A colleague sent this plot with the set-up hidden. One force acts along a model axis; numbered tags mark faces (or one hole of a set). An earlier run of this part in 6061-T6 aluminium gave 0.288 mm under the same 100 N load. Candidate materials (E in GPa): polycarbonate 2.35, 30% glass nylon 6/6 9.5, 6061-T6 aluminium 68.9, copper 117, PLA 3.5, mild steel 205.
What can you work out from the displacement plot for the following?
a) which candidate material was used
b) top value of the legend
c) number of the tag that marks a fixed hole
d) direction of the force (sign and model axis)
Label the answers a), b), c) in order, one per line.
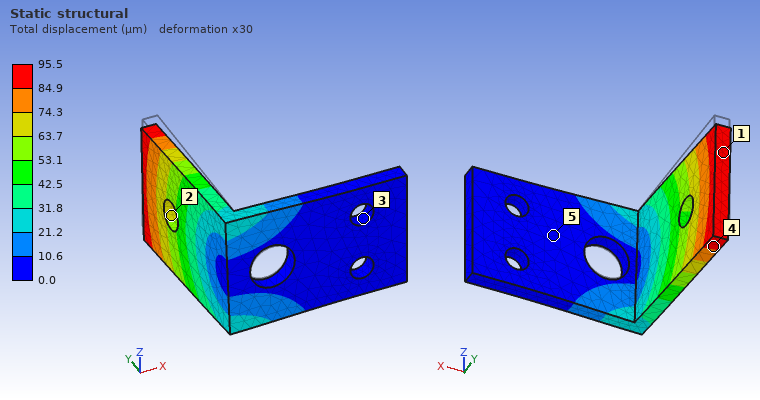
a) mild steel
b) 95.5 µm
c) 3
d) -Z
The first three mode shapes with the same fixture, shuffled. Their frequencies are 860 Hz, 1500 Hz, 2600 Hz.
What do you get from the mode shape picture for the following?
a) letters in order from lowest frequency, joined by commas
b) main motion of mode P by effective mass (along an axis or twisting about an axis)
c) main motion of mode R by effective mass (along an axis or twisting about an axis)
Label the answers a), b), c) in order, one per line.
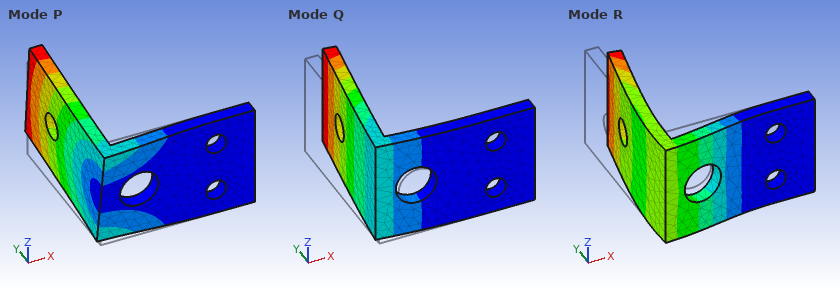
a) Q, P, R
b) along Z
c) along Y
